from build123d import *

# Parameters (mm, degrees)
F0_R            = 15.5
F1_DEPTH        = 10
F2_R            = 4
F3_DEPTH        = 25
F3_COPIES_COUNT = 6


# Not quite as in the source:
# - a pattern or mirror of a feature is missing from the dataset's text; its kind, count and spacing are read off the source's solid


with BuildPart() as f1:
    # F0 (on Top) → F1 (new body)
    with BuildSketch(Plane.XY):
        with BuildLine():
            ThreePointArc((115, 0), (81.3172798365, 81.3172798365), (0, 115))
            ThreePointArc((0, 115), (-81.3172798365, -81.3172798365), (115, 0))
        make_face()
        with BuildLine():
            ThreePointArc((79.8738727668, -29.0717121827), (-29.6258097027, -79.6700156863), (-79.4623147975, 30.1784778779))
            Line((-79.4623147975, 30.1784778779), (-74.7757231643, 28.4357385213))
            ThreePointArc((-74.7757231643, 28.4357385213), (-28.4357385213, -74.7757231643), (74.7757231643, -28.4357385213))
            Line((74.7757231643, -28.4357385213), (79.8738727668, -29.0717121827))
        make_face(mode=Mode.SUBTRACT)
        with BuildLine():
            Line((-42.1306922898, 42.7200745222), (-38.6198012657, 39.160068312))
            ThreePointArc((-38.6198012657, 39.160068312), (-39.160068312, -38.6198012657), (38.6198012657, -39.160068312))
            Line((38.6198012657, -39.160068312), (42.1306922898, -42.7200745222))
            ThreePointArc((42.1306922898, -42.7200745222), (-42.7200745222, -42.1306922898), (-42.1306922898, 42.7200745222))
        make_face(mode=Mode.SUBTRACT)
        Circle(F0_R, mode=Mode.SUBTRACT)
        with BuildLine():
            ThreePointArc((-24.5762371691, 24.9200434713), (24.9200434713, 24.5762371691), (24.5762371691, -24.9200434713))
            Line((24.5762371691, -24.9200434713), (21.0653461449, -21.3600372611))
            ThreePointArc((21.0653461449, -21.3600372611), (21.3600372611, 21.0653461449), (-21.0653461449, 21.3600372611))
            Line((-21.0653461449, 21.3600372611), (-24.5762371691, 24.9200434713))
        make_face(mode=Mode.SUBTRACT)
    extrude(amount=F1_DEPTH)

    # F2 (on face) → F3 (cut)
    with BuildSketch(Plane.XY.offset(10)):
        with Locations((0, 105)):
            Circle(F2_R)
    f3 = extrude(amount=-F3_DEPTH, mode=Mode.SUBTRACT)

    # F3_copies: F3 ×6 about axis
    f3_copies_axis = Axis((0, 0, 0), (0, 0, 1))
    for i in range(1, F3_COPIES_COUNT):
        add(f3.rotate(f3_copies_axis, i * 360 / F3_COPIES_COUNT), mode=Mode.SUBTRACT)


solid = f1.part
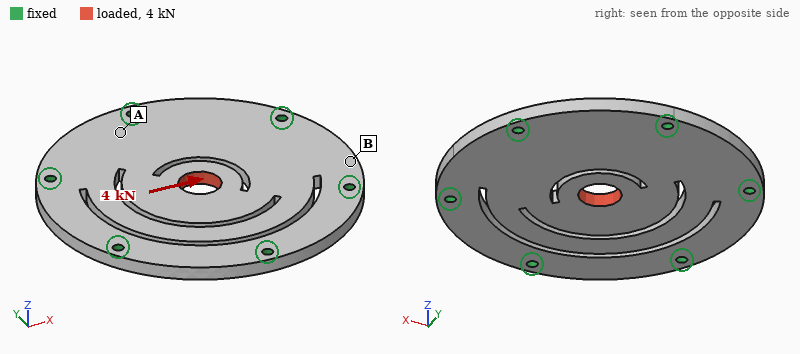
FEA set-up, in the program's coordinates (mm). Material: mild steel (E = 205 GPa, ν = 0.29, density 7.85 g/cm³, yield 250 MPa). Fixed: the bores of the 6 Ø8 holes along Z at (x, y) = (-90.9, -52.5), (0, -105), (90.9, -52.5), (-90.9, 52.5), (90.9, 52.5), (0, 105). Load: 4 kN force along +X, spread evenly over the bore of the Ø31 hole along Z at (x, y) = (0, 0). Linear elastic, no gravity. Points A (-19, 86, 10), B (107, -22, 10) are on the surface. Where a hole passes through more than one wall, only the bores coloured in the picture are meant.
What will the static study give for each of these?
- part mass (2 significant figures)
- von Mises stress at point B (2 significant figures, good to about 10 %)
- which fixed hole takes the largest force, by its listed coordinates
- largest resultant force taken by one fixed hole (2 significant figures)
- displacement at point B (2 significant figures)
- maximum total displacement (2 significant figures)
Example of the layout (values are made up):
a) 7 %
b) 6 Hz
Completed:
a) 3.0 kg
b) 5.5 MPa
c) (90.9, 52.5)
d) 1.4 kN
e) 1.9 µm
f) 9.4 µm
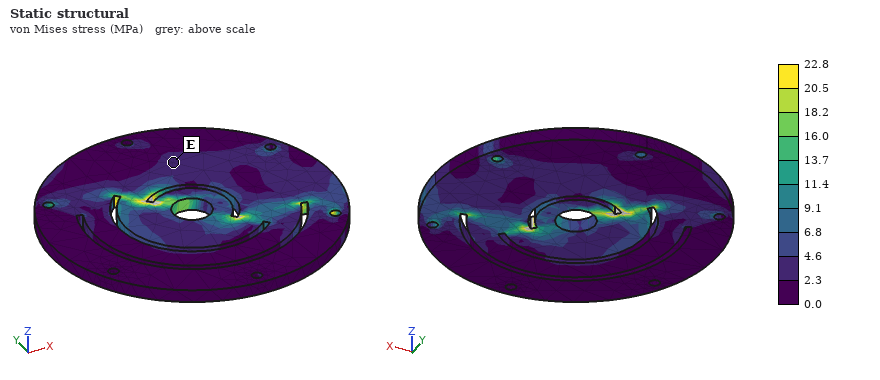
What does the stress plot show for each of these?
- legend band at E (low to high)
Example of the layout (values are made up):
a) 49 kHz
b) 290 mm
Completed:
a) 2.3 to 4.6 MPa
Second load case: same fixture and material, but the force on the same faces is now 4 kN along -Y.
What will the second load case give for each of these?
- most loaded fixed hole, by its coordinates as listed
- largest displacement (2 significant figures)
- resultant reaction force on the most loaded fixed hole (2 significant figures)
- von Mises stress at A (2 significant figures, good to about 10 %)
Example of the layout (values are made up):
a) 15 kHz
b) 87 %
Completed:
a) (0, 105)
b) 8.6 µm
c) 1.9 kN
d) 5.1 MPa
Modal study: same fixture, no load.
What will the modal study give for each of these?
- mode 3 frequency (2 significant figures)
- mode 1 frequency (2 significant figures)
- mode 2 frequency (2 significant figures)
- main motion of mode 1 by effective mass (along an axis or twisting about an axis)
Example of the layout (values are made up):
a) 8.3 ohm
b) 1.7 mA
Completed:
a) 1800 Hz
b) 590 Hz
c) 1000 Hz
d) along Z
